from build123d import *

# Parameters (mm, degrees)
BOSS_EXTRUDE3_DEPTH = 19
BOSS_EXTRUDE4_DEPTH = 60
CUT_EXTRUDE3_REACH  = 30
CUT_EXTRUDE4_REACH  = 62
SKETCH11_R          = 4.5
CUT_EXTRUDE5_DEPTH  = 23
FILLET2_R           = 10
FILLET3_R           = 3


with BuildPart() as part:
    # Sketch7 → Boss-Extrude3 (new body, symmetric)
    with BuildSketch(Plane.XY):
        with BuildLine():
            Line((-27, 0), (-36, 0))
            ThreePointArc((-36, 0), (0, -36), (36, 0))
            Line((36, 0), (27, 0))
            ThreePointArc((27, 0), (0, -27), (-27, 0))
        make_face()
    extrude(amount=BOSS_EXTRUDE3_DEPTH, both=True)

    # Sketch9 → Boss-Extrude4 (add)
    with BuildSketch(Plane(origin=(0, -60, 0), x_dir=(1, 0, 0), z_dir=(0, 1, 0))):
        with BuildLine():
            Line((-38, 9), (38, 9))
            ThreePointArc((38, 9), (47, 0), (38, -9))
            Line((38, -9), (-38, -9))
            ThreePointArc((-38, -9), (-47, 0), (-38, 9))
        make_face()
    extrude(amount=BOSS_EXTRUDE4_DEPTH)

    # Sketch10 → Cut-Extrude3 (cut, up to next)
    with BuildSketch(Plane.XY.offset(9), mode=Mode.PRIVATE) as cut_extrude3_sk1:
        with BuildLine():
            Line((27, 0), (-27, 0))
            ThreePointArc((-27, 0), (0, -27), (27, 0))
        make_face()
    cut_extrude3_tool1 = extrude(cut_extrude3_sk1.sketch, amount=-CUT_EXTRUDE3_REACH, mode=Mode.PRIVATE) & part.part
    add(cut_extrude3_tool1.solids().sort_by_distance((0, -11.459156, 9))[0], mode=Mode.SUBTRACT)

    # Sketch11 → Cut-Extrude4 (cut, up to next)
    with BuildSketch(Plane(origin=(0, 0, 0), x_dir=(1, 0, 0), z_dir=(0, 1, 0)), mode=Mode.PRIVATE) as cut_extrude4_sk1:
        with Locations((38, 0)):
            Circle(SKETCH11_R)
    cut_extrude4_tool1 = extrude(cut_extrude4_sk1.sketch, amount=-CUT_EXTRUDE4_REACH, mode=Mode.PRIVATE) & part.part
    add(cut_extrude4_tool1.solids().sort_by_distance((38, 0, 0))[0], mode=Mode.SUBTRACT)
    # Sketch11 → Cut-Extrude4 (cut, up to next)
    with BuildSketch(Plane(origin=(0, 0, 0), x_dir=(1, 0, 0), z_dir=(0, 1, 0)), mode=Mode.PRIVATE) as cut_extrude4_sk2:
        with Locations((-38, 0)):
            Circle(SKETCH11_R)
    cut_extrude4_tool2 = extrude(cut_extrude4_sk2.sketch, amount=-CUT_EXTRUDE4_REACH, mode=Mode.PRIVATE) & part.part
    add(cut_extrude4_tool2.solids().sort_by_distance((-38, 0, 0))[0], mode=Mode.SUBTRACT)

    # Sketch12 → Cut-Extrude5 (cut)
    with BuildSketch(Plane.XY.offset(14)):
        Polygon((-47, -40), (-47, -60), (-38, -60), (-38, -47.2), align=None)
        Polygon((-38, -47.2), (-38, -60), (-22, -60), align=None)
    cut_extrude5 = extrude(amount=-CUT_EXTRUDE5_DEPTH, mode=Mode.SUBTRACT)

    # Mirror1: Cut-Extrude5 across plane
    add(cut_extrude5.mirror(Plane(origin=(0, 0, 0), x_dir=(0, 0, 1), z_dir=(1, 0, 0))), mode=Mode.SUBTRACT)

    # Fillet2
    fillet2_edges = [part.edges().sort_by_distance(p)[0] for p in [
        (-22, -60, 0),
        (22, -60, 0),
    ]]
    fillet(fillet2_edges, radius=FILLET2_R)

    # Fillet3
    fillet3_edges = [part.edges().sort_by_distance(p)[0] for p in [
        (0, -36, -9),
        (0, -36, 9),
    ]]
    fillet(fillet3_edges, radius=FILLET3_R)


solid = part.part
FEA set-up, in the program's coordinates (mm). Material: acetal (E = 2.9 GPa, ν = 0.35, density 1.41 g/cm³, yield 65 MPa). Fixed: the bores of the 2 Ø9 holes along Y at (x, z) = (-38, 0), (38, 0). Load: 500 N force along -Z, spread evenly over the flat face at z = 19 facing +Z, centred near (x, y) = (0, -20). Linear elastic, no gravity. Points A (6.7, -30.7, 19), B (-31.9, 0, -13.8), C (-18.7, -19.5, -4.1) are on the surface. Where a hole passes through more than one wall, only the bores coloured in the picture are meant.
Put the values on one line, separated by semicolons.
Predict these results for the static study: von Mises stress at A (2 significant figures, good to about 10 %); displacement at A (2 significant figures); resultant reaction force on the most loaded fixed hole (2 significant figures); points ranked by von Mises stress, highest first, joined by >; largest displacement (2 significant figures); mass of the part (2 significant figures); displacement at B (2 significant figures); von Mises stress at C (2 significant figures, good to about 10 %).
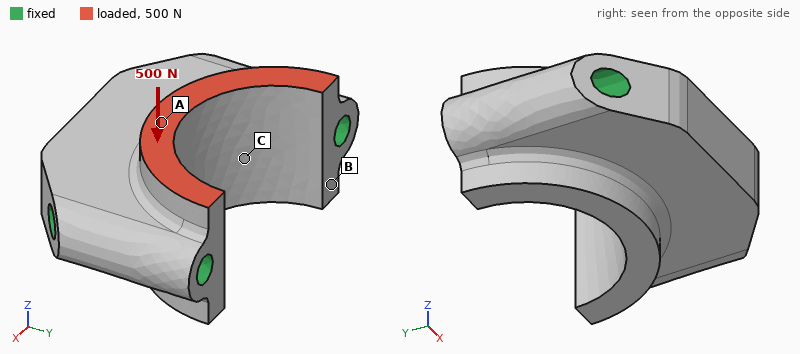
0.67 MPa; 11 µm; 250 N; A > C > B; 12 µm; 110 g; 2.8 µm; 0.37 MPa
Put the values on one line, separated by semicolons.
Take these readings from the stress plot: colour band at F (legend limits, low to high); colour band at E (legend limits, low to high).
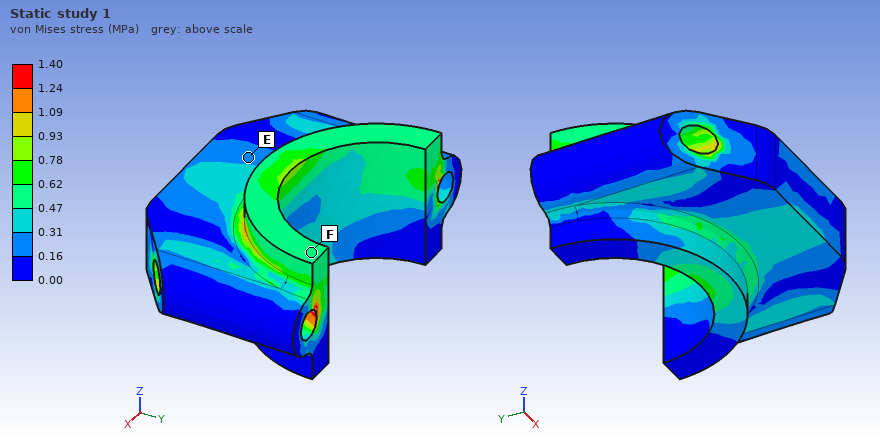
0.47 to 0.62 MPa; 0.16 to 0.31 MPa
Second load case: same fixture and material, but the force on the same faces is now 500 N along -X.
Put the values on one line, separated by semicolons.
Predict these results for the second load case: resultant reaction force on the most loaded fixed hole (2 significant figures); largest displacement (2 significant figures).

270 N; 30 µm
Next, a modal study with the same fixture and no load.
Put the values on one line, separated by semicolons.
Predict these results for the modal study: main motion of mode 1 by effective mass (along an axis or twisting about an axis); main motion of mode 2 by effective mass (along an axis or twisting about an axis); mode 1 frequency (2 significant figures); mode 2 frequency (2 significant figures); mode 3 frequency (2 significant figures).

along Z; along Y; 3300 Hz; 5300 Hz; 5600 Hz
